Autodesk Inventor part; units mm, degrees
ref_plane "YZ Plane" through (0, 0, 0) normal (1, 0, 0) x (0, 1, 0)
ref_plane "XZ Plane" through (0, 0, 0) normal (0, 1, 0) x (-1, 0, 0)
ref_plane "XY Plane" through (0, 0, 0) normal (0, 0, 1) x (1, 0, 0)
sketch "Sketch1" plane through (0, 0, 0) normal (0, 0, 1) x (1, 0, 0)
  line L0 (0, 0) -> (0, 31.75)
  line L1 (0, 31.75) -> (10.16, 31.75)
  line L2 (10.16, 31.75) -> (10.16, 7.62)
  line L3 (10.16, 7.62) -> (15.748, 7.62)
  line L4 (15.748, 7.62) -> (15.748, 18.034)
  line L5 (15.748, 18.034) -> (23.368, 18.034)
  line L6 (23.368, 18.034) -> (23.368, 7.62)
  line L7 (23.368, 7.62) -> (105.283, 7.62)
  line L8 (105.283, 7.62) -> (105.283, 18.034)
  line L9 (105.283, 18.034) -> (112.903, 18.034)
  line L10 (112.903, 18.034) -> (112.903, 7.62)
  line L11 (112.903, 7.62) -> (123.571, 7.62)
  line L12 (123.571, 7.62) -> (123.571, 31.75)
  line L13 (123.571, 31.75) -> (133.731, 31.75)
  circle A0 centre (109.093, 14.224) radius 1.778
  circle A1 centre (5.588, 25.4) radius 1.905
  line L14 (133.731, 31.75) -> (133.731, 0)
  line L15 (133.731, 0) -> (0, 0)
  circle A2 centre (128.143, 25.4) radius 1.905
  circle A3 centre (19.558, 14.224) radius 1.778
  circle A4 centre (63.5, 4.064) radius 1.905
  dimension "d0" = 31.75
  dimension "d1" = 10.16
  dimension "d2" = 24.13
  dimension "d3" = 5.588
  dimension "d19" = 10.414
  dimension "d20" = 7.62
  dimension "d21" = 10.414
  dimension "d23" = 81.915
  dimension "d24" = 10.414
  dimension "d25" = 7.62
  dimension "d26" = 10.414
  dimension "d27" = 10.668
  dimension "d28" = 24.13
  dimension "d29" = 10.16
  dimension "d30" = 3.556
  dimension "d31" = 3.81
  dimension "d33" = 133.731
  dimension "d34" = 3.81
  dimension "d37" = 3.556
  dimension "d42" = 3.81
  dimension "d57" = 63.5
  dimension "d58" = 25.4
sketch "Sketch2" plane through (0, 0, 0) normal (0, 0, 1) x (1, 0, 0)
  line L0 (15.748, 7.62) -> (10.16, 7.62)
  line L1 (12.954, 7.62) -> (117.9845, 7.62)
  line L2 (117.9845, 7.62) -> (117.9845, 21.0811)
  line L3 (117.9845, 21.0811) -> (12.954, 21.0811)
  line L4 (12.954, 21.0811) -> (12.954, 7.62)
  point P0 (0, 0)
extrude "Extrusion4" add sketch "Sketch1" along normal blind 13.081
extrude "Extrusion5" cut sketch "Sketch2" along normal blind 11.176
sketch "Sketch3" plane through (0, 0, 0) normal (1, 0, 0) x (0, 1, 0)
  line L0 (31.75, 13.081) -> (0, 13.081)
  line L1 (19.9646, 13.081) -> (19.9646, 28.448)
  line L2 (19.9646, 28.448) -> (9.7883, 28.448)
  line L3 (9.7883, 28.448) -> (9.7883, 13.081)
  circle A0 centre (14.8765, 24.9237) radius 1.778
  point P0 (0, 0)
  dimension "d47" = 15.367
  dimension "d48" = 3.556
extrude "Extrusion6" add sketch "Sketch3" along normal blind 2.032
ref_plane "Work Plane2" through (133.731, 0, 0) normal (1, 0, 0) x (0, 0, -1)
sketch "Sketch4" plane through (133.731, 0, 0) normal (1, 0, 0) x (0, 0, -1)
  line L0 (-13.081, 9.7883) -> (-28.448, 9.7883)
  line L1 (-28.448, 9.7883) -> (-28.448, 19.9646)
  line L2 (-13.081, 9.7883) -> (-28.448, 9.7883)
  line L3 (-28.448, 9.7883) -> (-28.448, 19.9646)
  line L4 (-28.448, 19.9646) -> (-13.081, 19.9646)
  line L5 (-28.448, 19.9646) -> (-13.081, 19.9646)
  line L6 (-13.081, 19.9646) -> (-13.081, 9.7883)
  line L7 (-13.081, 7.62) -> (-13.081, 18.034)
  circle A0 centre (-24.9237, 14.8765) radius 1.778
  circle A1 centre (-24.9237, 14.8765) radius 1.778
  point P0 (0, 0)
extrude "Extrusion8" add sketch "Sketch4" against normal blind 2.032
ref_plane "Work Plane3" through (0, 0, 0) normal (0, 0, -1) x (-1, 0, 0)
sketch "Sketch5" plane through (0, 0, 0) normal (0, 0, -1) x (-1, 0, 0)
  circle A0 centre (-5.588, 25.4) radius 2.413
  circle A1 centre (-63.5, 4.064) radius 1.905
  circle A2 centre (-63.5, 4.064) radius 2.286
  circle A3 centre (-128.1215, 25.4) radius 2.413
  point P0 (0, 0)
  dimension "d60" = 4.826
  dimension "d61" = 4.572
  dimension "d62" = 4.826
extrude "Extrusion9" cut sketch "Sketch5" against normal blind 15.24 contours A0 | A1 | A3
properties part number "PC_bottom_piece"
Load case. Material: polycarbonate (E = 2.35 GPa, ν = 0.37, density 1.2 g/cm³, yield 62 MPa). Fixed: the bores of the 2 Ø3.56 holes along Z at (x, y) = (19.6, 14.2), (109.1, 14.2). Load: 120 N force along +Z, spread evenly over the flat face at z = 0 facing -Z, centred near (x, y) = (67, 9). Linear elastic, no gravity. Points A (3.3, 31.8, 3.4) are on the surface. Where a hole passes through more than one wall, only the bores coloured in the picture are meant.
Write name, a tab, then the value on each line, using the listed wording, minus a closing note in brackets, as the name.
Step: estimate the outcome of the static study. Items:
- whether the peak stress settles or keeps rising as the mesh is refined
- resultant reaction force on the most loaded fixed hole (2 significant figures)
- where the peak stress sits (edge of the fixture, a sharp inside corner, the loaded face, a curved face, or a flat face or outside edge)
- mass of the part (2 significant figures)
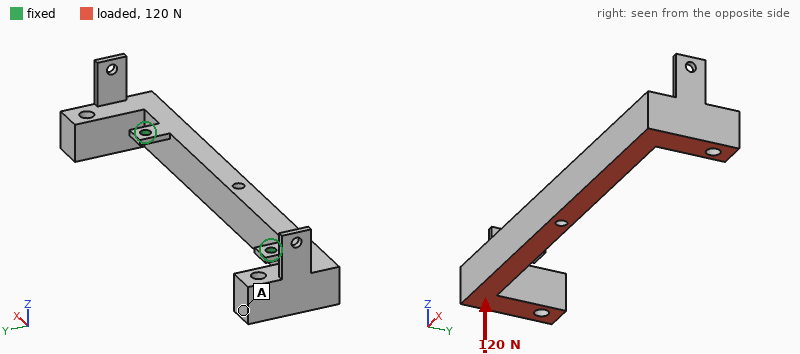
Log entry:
whether the peak stress settles or keeps rising as the mesh is refined	keeps rising
resultant reaction force on the most loaded fixed hole	63 N
where the peak stress sits	edge of the fixture
mass of the part	24 g
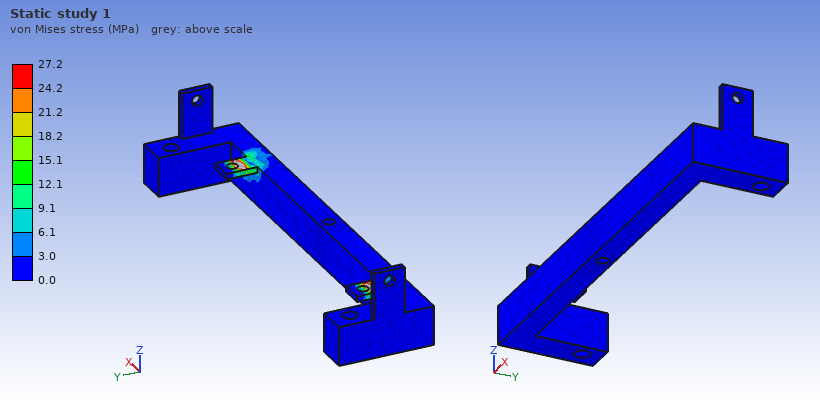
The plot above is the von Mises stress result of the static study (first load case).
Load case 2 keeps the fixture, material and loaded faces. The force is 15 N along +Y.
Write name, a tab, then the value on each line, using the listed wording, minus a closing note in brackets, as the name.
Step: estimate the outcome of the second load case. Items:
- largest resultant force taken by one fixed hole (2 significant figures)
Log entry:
largest resultant force taken by one fixed hole	7.9 N
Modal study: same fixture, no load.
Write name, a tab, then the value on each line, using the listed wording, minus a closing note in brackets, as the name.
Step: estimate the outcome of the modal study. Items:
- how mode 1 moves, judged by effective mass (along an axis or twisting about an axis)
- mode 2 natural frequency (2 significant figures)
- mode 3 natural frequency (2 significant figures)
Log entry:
how mode 1 moves, judged by effective mass	along Y
mode 2 natural frequency	540 Hz
mode 3 natural frequency	630 Hz
